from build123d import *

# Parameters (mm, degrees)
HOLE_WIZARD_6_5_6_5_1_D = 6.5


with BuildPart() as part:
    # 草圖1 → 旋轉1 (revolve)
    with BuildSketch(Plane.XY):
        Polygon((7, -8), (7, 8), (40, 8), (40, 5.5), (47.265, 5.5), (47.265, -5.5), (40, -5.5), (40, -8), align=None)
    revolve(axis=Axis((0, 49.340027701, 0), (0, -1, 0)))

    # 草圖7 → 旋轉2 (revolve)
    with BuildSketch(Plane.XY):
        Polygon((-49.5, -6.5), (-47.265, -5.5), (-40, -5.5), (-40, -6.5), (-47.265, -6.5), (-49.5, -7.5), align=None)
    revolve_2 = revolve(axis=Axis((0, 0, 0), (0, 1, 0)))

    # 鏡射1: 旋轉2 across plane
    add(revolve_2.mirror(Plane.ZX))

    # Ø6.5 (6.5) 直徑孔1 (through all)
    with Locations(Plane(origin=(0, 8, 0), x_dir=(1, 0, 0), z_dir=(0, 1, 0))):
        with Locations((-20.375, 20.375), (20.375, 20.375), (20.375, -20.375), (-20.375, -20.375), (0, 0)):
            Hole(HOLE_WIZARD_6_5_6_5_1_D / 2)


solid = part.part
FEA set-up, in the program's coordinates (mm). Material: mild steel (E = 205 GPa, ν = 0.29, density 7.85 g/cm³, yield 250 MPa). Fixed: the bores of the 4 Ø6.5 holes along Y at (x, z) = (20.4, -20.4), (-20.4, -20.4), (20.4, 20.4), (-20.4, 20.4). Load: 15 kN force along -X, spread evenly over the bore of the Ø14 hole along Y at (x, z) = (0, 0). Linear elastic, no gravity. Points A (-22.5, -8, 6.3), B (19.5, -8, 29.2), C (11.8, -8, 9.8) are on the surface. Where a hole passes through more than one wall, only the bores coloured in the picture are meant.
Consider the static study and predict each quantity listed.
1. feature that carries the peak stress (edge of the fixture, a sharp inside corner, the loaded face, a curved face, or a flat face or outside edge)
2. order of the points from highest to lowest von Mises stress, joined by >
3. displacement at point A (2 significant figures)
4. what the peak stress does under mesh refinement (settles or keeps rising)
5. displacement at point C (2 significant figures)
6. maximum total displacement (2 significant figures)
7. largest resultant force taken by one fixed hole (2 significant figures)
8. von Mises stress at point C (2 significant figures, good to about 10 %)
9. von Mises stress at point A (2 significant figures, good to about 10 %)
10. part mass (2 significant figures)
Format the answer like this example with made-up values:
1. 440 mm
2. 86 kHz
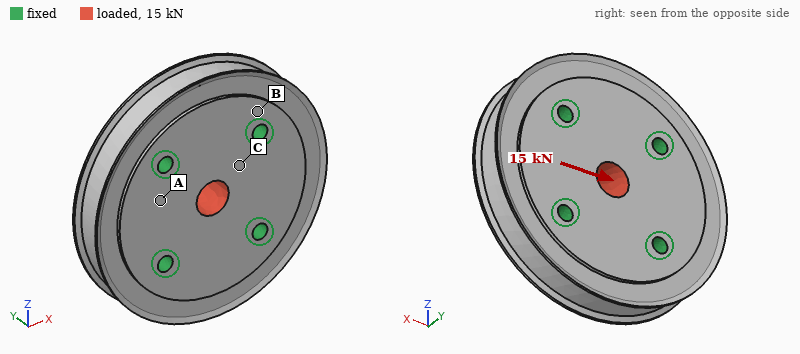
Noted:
1. edge of the fixture
2. C > A > B
3. 0.99 µm
4. keeps rising
5. 1.1 µm
6. 2.2 µm
7. 3.9 kN
8. 15 MPa
9. 7.9 MPa
10. 810 g
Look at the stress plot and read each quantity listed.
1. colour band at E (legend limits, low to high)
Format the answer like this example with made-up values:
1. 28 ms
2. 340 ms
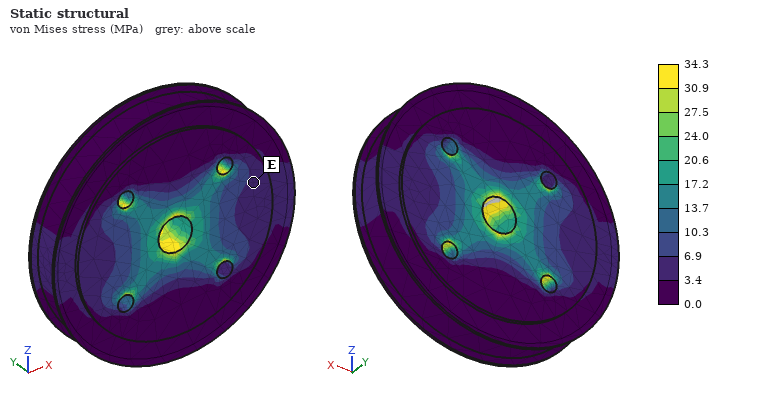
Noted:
1. 3.4 to 6.9 MPa
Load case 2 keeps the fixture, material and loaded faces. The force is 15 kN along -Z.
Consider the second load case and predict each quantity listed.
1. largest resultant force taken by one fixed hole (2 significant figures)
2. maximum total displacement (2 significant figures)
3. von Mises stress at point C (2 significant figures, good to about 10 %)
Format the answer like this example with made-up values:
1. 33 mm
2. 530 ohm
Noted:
1. 3.9 kN
2. 2.2 µm
3. 15 MPa
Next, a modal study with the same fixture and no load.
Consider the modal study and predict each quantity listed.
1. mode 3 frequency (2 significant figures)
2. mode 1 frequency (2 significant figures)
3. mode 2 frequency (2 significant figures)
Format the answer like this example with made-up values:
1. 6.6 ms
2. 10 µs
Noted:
1. 16 kHz
2. 15 kHz
3. 16 kHz
